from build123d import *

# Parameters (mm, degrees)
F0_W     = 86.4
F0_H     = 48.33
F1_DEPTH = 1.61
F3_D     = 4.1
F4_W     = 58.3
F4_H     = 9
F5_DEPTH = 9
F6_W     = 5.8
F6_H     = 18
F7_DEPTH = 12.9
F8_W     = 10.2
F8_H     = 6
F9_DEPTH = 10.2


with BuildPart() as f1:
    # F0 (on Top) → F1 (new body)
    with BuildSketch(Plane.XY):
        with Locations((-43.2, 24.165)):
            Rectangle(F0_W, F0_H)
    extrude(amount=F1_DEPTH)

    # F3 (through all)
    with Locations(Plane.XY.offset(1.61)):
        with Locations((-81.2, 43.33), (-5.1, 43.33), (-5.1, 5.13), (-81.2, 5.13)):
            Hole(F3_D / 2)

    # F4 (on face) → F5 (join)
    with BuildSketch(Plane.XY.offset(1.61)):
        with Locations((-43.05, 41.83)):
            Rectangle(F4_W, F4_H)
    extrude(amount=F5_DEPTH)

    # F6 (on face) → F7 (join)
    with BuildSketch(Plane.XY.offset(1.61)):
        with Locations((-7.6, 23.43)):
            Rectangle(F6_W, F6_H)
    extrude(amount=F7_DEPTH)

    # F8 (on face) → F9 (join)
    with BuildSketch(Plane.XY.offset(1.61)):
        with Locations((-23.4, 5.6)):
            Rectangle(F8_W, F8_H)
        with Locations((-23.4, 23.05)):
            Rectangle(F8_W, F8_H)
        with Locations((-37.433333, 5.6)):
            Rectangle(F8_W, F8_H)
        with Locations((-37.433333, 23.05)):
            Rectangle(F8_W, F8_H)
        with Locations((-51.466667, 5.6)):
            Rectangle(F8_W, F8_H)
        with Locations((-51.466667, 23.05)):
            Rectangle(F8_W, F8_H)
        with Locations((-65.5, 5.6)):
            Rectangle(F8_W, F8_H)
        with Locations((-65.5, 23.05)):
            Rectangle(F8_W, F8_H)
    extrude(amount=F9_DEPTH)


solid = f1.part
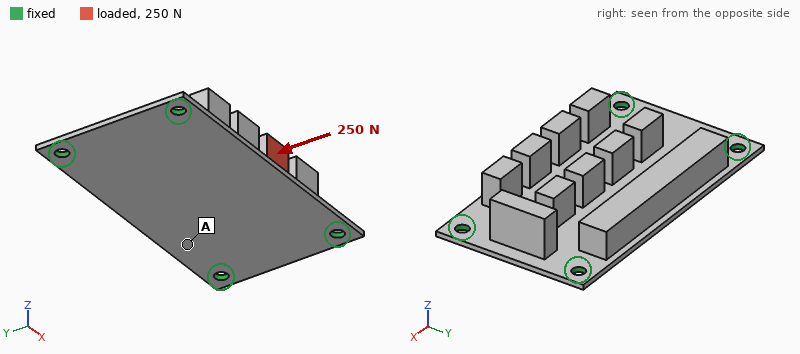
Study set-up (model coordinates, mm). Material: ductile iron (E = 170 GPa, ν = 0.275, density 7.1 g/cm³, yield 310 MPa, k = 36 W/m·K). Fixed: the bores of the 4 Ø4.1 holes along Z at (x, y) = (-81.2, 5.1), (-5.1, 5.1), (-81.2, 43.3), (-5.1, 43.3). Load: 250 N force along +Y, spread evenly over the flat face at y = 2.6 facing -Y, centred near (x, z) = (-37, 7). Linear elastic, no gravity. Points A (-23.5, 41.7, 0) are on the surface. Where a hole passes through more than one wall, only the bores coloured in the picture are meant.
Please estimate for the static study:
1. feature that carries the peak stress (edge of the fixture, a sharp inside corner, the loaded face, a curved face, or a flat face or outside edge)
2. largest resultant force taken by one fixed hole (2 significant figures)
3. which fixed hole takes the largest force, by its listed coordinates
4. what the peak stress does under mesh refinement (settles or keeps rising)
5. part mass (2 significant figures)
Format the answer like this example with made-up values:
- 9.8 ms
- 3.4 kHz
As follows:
- edge of the fixture
- 110 N
- (-5.1, 43.3)
- keeps rising
- 130 g
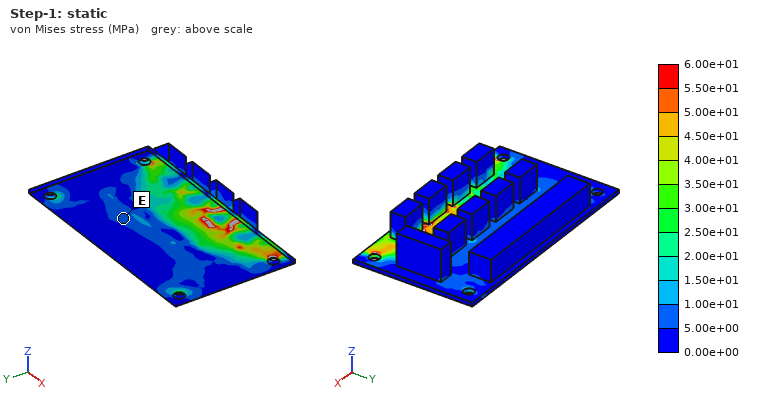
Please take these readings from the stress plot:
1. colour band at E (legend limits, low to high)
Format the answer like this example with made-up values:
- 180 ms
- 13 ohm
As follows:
- 5.00e+00 to 1.00e+01 MPa
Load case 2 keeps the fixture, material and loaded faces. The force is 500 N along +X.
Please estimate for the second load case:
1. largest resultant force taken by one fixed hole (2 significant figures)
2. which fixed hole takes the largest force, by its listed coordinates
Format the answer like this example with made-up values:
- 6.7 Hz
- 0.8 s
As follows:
- 210 N
- (-5.1, 5.1)
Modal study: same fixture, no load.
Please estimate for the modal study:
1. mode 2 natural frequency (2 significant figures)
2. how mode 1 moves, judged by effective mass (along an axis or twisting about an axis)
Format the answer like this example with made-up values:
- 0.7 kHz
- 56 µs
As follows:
- 2400 Hz
- along Z
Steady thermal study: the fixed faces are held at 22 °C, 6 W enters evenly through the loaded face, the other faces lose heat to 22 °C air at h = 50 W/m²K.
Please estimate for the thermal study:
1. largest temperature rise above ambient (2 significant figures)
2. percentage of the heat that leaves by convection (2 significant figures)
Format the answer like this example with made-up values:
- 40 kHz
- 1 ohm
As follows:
- 52 K
- 75 %
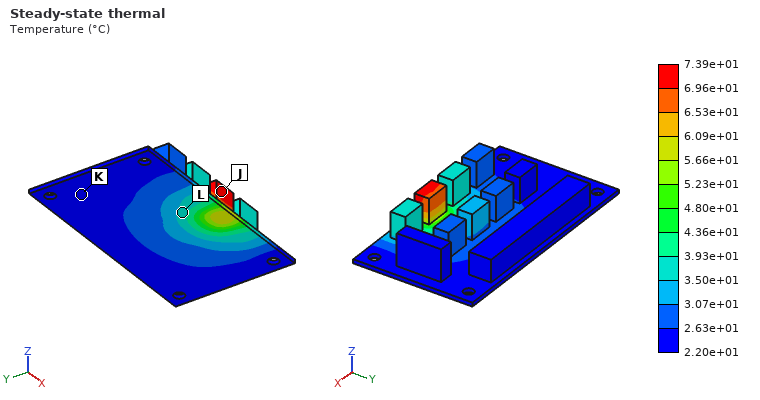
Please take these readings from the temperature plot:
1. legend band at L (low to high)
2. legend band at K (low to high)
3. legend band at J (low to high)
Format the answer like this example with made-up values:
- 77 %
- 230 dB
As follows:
- 3.50e+01 to 3.93e+01 °C
- 2.20e+01 to 2.63e+01 °C
- 6.96e+01 to 7.39e+01 °C
